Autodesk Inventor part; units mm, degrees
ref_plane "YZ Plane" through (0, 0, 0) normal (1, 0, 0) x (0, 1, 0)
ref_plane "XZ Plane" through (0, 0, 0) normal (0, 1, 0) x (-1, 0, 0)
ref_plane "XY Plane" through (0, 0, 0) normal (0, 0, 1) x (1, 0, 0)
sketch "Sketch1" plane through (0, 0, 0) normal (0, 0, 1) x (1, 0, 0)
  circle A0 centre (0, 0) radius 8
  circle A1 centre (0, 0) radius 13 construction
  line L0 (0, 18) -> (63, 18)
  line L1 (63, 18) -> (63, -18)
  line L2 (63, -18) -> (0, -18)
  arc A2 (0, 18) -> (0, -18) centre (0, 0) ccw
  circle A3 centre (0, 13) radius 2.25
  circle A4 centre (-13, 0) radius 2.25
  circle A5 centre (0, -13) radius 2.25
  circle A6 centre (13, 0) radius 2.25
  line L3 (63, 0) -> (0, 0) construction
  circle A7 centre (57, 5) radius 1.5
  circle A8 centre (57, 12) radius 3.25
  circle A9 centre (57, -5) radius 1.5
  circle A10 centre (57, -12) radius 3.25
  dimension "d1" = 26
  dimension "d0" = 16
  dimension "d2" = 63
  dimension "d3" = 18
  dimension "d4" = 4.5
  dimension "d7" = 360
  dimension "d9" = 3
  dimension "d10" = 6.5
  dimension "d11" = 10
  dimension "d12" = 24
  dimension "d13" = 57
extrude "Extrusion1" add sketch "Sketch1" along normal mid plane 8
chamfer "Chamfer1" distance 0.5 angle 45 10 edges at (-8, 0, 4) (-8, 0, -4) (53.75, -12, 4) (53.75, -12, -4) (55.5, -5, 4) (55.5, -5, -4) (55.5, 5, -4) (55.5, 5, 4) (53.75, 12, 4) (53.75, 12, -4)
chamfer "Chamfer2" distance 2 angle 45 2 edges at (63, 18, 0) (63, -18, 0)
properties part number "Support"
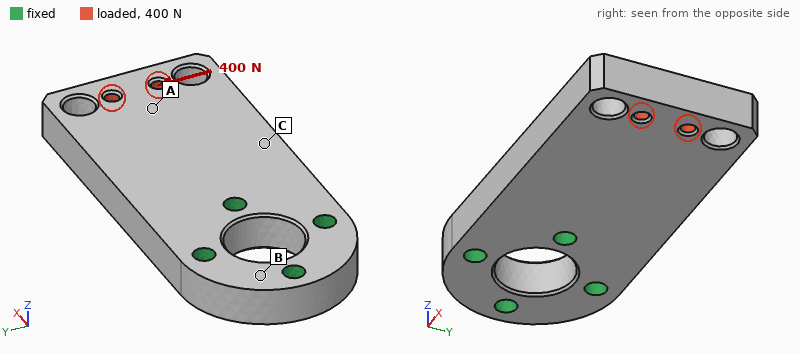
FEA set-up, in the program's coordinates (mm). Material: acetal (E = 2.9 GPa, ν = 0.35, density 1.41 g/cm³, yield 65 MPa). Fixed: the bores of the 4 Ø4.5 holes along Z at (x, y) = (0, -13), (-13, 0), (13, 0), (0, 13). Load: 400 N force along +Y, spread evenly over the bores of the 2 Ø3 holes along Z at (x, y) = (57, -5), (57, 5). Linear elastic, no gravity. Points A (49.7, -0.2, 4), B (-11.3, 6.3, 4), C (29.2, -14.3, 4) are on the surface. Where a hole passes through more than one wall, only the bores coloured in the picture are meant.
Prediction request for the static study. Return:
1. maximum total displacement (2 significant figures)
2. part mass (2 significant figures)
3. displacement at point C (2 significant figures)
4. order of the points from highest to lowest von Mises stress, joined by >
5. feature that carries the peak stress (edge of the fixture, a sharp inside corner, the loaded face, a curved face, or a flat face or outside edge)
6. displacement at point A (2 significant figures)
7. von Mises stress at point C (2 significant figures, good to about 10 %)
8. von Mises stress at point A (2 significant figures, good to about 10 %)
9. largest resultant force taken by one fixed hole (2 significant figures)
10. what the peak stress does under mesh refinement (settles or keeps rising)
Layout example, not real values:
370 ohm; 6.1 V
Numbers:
0.36 mm; 27 g; 0.11 mm; C > A > B; edge of the fixture; 0.24 mm; 5.4 MPa; 3.4 MPa; 570 N; keeps rising
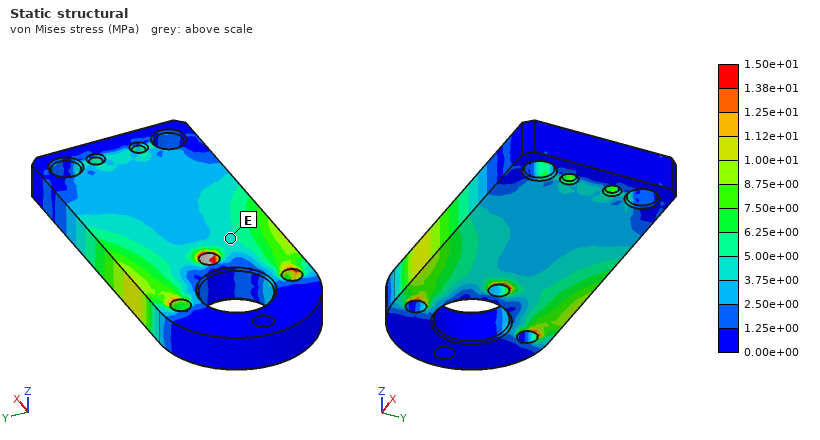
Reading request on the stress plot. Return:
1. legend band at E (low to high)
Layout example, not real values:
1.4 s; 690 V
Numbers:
3.75e+00 to 5.00e+00 MPa
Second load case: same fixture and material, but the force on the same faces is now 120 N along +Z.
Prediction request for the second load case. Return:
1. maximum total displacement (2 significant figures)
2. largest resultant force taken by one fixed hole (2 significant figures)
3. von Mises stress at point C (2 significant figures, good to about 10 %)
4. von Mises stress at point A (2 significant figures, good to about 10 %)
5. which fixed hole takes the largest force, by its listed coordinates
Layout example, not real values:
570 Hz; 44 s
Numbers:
1.0 mm; 280 N; 8.4 MPa; 3.1 MPa; (13, 0)
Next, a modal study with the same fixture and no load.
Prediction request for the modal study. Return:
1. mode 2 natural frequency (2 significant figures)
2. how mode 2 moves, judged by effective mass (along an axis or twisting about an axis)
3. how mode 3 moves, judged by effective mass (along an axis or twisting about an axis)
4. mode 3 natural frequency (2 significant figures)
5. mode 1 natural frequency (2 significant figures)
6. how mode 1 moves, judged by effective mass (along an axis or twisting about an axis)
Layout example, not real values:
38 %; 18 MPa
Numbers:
1800 Hz; twisting about X; along Y; 2100 Hz; 740 Hz; along Z
